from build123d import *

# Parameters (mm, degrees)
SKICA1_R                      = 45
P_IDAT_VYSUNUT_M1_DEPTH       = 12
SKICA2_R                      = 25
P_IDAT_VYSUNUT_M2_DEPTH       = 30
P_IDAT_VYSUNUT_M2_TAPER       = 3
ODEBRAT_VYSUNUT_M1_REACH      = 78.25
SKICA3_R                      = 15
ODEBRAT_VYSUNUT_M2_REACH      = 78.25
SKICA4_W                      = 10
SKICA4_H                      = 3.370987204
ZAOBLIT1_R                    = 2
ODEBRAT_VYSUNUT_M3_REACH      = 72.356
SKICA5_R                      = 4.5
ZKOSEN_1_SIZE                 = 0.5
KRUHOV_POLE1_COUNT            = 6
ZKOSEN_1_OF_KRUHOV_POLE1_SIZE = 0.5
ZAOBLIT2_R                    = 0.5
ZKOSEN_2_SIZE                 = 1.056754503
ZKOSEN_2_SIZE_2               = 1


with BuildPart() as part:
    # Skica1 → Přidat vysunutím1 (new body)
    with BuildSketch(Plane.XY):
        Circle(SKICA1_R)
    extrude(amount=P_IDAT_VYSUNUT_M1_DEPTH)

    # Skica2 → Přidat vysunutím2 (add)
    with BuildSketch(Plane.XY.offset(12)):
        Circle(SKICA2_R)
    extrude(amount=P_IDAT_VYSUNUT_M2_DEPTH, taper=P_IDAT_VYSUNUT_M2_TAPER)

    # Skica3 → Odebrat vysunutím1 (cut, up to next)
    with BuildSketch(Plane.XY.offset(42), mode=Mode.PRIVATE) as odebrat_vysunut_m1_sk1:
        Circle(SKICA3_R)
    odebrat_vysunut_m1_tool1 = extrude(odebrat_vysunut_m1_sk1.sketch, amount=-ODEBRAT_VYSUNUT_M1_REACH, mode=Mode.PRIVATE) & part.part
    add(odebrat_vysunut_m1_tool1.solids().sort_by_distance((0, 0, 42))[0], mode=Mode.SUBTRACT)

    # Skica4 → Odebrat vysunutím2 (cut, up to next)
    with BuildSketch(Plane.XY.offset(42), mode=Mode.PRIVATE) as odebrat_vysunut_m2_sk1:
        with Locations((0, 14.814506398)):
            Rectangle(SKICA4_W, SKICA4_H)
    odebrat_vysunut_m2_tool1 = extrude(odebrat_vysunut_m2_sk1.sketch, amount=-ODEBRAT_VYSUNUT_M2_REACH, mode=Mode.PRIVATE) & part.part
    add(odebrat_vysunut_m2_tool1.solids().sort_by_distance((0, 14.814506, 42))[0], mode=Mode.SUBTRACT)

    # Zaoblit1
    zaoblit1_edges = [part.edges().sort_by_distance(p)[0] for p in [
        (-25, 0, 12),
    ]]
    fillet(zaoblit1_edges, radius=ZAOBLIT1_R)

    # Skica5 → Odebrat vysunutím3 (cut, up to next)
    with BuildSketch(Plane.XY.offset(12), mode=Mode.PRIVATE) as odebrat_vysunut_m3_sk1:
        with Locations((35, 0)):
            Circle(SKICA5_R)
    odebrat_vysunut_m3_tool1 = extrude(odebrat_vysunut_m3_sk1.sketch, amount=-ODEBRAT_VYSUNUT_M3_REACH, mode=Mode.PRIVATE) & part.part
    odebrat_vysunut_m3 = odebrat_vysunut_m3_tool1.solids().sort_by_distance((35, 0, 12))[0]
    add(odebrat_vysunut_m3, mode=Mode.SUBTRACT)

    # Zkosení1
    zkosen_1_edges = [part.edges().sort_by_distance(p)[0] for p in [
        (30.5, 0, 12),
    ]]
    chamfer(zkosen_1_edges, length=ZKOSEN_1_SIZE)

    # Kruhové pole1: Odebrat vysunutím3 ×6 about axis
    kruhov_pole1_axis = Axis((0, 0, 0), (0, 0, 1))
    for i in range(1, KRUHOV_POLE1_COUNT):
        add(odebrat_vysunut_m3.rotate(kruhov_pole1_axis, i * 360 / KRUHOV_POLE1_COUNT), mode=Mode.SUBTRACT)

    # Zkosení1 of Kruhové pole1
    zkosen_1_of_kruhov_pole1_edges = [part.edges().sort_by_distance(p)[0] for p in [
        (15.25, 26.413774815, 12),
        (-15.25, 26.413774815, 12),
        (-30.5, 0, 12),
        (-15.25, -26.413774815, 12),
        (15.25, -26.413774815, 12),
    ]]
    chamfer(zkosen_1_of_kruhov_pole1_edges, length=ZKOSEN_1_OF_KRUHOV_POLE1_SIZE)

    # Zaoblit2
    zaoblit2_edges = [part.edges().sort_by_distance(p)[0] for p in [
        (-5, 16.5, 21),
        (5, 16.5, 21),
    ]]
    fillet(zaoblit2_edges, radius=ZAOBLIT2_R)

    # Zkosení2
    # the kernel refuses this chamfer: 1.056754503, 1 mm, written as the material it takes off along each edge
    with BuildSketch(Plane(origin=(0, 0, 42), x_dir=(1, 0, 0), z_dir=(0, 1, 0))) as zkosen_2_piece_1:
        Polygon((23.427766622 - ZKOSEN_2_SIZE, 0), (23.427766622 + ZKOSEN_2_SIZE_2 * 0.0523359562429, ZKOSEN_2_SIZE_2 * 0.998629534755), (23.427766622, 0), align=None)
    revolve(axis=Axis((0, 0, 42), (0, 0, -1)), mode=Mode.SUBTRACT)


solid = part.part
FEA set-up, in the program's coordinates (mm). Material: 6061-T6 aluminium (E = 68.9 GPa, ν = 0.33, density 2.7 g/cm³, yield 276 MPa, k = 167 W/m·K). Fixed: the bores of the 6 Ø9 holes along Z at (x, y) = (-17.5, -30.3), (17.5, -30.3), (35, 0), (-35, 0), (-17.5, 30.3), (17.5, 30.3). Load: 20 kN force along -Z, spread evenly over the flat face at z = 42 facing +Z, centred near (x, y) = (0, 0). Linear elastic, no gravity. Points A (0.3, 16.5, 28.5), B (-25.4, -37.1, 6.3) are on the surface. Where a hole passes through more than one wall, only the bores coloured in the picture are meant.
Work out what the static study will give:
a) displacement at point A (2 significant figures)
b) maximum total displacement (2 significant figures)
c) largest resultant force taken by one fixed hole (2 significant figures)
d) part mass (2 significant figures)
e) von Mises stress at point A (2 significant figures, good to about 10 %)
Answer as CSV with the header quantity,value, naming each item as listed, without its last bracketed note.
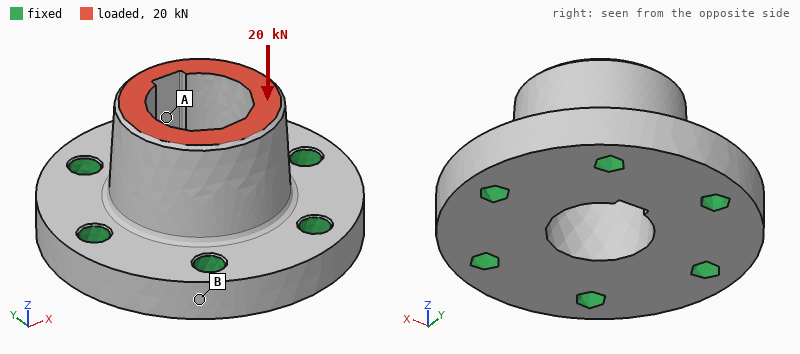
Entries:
quantity,value
displacement at point A,12 µm
maximum total displacement,17 µm
largest resultant force taken by one fixed hole,3.7 kN
part mass,260 g
von Mises stress at point A,21 MPa
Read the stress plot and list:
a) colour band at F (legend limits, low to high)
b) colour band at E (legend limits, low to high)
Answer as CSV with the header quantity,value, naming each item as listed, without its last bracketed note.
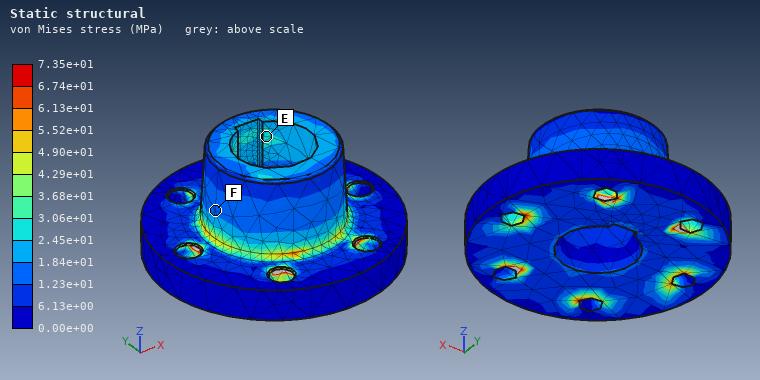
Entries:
quantity,value
colour band at F,1.23e+01 to 1.84e+01 MPa
colour band at E,2.45e+01 to 3.06e+01 MPa
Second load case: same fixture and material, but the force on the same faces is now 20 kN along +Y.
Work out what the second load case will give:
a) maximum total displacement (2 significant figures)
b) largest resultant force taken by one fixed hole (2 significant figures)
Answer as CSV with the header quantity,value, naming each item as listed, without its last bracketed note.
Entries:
quantity,value
maximum total displacement,91 µm
largest resultant force taken by one fixed hole,8.2 kN
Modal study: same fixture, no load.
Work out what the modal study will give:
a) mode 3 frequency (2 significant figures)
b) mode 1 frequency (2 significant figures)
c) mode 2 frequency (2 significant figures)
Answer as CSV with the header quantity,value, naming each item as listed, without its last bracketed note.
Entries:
quantity,value
mode 3 frequency,18 kHz
mode 1 frequency,14 kHz
mode 2 frequency,14 kHz
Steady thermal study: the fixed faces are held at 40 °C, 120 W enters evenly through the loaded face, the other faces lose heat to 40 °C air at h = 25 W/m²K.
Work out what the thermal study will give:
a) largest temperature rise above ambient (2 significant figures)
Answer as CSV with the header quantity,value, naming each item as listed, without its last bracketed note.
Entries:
quantity,value
largest temperature rise above ambient,26 K
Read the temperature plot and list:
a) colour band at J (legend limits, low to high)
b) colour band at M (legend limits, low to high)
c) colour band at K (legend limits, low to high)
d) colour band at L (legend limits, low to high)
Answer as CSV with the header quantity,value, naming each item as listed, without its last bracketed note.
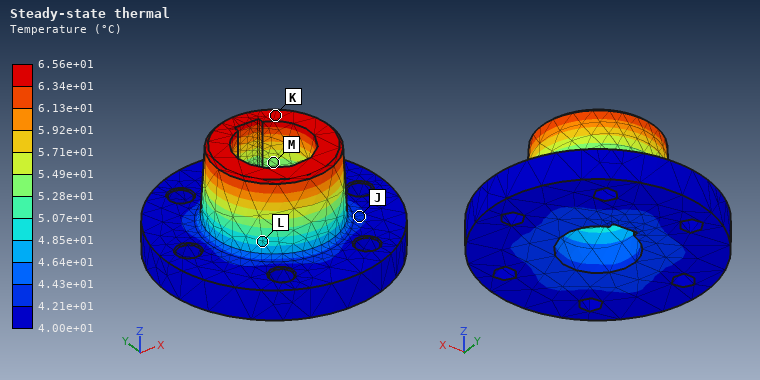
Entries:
quantity,value
colour band at J,4.21e+01 to 4.43e+01 °C
colour band at M,5.28e+01 to 5.49e+01 °C
colour band at K,6.34e+01 to 6.56e+01 °C
colour band at L,4.85e+01 to 5.07e+01 °C
